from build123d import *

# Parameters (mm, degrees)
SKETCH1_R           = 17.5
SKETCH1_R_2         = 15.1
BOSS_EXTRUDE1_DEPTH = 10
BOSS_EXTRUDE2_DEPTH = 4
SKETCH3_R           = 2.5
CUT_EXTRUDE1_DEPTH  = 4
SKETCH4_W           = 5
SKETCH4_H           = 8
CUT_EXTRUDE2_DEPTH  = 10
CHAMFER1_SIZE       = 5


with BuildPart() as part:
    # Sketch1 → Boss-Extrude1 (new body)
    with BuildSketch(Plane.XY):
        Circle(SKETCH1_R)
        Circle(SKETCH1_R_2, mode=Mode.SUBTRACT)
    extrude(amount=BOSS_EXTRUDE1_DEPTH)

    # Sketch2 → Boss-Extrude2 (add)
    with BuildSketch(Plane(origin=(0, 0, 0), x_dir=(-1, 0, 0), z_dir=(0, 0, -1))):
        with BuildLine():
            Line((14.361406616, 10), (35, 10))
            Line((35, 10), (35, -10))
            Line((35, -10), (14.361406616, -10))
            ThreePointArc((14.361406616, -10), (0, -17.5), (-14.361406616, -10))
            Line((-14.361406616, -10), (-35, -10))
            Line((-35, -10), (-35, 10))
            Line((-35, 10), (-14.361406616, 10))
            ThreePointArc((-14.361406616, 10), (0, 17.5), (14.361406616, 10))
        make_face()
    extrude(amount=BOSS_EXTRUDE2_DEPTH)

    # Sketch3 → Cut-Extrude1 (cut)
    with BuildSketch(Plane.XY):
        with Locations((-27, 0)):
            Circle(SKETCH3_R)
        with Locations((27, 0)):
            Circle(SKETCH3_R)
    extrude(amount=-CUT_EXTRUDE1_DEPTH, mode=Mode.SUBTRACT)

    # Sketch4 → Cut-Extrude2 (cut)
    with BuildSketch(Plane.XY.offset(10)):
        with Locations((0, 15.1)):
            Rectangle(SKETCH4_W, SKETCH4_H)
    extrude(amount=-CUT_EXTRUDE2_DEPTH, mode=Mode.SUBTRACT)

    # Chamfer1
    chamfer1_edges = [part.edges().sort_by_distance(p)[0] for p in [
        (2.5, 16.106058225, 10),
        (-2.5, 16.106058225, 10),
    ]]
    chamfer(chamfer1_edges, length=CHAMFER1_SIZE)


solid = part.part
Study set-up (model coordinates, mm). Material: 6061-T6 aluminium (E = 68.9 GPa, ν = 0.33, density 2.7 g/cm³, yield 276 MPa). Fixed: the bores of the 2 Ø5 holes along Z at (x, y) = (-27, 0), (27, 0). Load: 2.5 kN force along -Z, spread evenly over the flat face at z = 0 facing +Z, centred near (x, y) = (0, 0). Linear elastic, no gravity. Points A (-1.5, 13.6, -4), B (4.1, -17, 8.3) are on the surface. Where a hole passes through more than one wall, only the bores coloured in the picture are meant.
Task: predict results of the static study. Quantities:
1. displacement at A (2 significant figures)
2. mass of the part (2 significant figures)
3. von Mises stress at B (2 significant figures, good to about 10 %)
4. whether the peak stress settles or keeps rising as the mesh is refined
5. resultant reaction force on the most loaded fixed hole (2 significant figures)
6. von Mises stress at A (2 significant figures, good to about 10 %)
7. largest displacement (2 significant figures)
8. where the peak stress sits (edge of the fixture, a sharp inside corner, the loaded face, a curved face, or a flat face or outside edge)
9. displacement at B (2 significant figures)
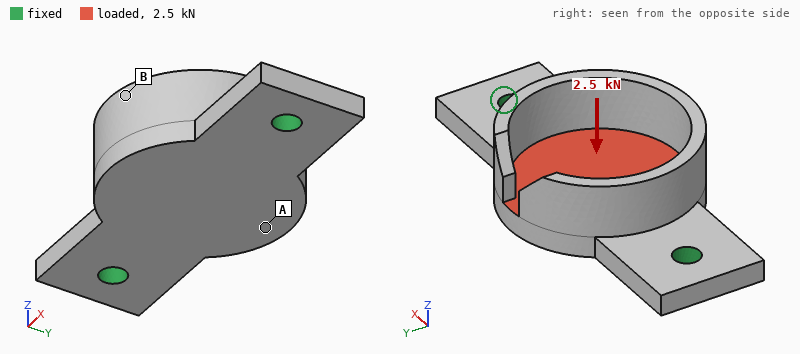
0.17 mm
24 g
35 MPa
keeps rising
1.3 kN
120 MPa
0.19 mm
edge of the fixture
0.14 mm
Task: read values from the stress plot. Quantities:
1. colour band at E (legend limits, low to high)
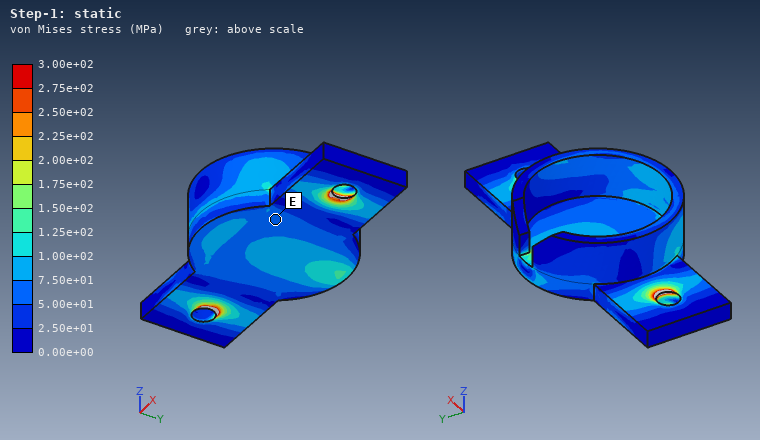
5.00e+01 to 7.50e+01 MPa
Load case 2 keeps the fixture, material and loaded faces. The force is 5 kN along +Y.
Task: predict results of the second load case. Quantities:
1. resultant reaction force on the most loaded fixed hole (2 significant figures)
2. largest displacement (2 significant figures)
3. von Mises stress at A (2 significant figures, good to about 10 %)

2.5 kN
0.12 mm
43 MPa
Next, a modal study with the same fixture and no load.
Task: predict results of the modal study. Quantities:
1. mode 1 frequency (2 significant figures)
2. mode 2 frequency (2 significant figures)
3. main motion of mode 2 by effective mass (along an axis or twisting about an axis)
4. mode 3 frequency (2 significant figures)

5100 Hz
5700 Hz
along Z
14 kHz
